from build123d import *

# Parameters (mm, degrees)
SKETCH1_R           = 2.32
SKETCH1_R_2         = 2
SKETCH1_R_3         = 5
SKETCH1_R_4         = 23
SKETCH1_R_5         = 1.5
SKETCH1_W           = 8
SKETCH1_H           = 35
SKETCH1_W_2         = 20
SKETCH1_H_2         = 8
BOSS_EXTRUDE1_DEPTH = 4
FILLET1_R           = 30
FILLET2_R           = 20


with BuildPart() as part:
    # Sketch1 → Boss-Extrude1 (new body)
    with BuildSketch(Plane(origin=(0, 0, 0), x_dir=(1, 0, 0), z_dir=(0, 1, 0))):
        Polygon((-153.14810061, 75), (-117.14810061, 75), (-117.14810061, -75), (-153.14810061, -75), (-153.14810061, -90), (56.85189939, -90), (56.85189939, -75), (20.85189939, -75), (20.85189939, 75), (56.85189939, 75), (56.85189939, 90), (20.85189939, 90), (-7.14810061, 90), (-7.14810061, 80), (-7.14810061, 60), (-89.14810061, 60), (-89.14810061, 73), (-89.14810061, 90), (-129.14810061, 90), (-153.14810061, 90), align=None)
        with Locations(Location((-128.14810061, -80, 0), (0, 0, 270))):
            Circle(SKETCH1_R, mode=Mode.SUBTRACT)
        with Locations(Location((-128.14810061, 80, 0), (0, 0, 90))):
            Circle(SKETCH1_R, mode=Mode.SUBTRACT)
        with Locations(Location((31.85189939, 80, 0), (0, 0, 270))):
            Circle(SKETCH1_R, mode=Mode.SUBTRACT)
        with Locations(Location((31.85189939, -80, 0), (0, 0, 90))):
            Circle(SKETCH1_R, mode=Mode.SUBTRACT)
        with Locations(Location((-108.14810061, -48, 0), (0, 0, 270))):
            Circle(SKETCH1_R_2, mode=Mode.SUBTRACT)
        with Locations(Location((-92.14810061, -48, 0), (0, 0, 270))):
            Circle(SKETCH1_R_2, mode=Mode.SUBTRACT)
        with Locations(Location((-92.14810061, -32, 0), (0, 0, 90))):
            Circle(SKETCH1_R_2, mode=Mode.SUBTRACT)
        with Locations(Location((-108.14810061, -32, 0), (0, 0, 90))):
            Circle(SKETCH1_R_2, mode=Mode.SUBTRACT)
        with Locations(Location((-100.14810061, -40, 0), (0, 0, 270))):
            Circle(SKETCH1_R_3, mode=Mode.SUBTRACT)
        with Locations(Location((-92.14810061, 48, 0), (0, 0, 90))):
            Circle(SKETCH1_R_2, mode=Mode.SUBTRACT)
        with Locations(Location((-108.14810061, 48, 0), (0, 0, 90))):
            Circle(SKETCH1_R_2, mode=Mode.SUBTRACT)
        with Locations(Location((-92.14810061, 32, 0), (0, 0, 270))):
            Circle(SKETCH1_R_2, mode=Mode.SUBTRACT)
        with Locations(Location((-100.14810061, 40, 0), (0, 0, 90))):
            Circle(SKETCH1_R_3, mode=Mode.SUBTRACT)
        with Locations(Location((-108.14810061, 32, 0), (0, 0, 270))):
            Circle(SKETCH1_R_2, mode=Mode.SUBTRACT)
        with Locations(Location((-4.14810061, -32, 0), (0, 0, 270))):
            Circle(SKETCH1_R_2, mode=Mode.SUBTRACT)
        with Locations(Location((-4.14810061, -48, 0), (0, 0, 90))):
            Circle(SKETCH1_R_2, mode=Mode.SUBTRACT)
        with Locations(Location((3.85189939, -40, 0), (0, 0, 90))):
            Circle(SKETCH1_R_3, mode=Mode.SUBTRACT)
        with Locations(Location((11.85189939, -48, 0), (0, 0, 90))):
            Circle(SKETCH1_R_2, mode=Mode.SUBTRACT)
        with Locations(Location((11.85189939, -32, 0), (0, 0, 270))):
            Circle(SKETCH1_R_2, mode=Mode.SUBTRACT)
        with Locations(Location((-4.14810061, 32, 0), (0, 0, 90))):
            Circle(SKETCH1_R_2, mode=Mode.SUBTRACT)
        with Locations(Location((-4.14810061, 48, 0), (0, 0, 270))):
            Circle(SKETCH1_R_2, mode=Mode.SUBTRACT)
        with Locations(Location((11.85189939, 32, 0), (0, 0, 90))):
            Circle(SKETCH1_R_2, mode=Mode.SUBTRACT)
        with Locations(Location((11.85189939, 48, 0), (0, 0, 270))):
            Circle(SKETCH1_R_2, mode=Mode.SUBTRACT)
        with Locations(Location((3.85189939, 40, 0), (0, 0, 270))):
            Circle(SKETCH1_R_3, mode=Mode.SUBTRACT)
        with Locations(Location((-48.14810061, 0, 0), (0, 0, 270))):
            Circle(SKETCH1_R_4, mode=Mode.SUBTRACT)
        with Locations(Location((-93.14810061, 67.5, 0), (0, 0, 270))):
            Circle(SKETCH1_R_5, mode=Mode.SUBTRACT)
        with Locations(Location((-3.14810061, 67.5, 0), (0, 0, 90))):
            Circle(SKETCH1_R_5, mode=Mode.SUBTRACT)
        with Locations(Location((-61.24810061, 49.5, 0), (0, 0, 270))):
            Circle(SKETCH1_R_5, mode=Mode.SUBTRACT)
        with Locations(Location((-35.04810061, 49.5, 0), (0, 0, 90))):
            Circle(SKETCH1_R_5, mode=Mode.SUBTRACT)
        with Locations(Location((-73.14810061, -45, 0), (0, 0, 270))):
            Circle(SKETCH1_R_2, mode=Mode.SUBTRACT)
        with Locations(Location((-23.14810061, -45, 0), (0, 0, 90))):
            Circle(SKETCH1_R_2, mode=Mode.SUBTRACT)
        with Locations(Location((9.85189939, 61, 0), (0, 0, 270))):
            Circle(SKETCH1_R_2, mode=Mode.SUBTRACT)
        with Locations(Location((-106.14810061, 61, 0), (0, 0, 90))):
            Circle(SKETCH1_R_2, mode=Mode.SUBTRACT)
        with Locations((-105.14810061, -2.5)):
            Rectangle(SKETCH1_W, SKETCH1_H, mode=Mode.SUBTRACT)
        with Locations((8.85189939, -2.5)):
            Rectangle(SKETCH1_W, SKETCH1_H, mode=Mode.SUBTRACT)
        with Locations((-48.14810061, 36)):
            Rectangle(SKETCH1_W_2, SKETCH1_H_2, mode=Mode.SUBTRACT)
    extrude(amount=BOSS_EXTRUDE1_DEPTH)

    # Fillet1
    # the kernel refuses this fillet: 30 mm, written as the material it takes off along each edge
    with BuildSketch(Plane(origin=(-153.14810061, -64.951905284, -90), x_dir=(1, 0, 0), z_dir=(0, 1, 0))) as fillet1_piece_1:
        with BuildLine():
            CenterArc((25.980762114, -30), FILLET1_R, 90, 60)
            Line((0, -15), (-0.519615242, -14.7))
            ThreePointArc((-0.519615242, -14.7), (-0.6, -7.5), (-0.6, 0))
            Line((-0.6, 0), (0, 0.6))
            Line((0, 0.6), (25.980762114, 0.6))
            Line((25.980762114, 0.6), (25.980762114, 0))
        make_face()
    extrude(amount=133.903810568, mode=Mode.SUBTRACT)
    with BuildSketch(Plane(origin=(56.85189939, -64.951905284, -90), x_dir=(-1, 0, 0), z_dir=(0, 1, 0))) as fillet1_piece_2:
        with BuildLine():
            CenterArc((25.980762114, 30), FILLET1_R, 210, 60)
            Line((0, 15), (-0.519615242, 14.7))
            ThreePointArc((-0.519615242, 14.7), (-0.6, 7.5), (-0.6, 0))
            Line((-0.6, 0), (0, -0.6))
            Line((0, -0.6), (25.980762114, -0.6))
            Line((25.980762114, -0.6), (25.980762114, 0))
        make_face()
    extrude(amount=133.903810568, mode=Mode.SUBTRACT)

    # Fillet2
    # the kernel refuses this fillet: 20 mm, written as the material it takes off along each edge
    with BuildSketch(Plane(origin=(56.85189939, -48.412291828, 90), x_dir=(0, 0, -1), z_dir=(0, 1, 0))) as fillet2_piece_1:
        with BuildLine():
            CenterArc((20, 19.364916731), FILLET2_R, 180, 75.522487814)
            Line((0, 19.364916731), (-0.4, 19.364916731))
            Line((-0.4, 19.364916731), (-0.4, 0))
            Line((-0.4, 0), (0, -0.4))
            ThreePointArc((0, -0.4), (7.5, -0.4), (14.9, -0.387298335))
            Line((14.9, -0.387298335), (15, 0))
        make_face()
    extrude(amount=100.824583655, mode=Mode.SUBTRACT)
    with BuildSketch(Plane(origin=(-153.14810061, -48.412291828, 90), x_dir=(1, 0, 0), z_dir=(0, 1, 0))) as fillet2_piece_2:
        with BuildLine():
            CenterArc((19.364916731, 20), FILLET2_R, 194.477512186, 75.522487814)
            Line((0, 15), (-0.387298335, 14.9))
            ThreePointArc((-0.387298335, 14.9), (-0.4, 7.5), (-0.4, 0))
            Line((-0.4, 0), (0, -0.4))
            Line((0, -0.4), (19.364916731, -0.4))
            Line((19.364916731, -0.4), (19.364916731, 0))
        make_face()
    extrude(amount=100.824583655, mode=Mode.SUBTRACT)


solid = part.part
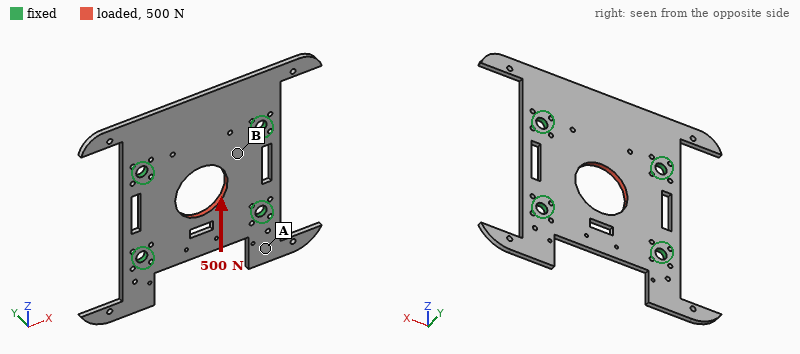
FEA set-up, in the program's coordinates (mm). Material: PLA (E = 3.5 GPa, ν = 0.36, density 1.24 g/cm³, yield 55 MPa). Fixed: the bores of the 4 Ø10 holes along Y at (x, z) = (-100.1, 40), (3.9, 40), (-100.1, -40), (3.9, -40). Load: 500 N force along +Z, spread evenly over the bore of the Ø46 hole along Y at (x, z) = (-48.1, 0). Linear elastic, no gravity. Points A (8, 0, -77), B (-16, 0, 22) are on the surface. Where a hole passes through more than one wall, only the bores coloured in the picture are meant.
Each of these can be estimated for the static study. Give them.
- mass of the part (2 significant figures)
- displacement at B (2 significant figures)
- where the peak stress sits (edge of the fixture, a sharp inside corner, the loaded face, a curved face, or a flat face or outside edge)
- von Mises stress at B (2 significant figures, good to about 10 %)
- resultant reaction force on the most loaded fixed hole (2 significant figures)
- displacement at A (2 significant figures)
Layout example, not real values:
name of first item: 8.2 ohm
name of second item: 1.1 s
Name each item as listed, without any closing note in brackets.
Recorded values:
mass of the part: 100 g
displacement at B: 11 µm
where the peak stress sits: a curved face
von Mises stress at B: 0.88 MPa
resultant reaction force on the most loaded fixed hole: 140 N
displacement at A: 14 µm
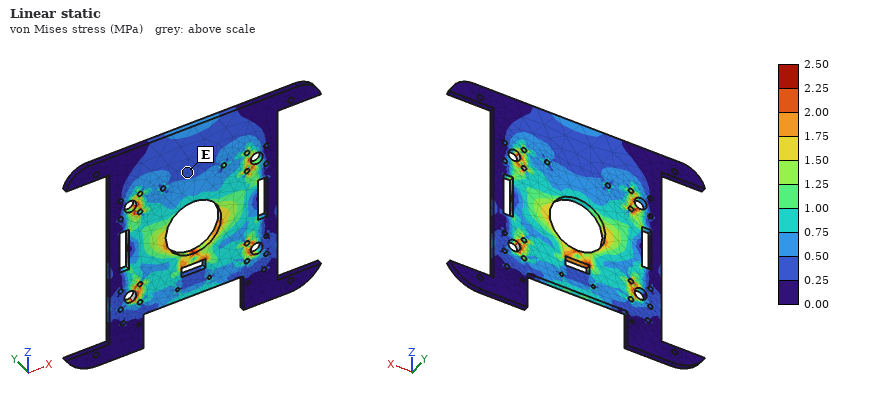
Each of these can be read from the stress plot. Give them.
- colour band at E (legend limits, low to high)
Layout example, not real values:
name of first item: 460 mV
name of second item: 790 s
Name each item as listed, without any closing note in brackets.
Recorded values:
colour band at E: 0.25 to 0.50 MPa
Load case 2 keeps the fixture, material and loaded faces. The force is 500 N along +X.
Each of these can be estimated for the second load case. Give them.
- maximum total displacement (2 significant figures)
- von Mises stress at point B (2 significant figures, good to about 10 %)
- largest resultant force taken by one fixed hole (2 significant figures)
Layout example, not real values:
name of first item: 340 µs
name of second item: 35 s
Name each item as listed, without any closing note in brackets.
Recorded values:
maximum total displacement: 19 µm
von Mises stress at point B: 0.98 MPa
largest resultant force taken by one fixed hole: 140 N
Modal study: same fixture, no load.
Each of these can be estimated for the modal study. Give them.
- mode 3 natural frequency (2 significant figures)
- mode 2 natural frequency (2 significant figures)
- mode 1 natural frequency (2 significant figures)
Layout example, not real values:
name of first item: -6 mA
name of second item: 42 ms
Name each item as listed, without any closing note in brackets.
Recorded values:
mode 3 natural frequency: 330 Hz
mode 2 natural frequency: 320 Hz
mode 1 natural frequency: 320 Hz
